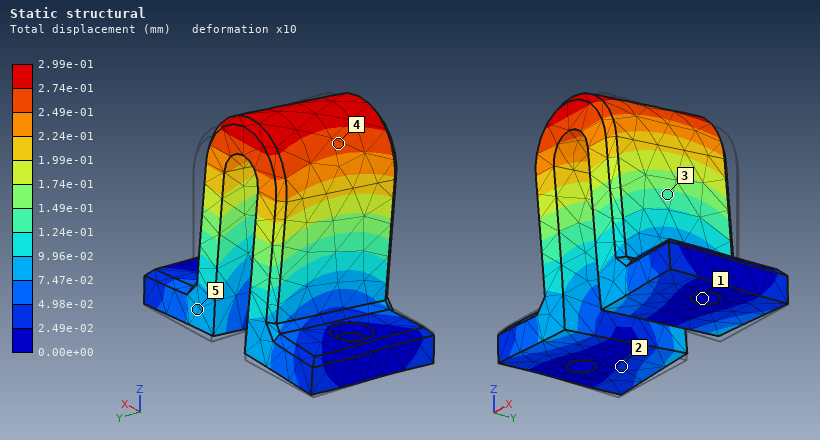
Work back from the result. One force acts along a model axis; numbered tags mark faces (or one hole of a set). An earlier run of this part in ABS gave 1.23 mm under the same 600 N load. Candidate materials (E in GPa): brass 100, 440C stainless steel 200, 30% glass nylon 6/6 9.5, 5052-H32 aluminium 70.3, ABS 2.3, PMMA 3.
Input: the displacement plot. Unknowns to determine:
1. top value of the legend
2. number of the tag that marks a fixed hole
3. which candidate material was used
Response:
2.99e-01 mm
1
30% glass nylon 6/6
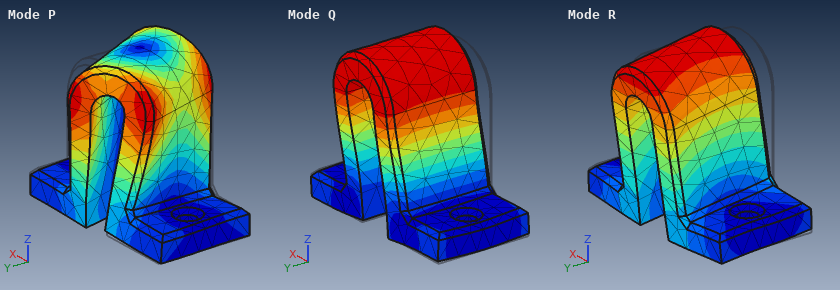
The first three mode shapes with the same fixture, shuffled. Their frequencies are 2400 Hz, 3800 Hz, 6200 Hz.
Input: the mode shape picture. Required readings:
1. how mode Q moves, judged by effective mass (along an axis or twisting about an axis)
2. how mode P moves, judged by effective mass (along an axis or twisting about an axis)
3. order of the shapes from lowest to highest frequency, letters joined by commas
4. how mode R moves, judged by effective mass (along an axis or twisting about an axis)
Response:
along X
twisting about Z
R, Q, P
along Y
